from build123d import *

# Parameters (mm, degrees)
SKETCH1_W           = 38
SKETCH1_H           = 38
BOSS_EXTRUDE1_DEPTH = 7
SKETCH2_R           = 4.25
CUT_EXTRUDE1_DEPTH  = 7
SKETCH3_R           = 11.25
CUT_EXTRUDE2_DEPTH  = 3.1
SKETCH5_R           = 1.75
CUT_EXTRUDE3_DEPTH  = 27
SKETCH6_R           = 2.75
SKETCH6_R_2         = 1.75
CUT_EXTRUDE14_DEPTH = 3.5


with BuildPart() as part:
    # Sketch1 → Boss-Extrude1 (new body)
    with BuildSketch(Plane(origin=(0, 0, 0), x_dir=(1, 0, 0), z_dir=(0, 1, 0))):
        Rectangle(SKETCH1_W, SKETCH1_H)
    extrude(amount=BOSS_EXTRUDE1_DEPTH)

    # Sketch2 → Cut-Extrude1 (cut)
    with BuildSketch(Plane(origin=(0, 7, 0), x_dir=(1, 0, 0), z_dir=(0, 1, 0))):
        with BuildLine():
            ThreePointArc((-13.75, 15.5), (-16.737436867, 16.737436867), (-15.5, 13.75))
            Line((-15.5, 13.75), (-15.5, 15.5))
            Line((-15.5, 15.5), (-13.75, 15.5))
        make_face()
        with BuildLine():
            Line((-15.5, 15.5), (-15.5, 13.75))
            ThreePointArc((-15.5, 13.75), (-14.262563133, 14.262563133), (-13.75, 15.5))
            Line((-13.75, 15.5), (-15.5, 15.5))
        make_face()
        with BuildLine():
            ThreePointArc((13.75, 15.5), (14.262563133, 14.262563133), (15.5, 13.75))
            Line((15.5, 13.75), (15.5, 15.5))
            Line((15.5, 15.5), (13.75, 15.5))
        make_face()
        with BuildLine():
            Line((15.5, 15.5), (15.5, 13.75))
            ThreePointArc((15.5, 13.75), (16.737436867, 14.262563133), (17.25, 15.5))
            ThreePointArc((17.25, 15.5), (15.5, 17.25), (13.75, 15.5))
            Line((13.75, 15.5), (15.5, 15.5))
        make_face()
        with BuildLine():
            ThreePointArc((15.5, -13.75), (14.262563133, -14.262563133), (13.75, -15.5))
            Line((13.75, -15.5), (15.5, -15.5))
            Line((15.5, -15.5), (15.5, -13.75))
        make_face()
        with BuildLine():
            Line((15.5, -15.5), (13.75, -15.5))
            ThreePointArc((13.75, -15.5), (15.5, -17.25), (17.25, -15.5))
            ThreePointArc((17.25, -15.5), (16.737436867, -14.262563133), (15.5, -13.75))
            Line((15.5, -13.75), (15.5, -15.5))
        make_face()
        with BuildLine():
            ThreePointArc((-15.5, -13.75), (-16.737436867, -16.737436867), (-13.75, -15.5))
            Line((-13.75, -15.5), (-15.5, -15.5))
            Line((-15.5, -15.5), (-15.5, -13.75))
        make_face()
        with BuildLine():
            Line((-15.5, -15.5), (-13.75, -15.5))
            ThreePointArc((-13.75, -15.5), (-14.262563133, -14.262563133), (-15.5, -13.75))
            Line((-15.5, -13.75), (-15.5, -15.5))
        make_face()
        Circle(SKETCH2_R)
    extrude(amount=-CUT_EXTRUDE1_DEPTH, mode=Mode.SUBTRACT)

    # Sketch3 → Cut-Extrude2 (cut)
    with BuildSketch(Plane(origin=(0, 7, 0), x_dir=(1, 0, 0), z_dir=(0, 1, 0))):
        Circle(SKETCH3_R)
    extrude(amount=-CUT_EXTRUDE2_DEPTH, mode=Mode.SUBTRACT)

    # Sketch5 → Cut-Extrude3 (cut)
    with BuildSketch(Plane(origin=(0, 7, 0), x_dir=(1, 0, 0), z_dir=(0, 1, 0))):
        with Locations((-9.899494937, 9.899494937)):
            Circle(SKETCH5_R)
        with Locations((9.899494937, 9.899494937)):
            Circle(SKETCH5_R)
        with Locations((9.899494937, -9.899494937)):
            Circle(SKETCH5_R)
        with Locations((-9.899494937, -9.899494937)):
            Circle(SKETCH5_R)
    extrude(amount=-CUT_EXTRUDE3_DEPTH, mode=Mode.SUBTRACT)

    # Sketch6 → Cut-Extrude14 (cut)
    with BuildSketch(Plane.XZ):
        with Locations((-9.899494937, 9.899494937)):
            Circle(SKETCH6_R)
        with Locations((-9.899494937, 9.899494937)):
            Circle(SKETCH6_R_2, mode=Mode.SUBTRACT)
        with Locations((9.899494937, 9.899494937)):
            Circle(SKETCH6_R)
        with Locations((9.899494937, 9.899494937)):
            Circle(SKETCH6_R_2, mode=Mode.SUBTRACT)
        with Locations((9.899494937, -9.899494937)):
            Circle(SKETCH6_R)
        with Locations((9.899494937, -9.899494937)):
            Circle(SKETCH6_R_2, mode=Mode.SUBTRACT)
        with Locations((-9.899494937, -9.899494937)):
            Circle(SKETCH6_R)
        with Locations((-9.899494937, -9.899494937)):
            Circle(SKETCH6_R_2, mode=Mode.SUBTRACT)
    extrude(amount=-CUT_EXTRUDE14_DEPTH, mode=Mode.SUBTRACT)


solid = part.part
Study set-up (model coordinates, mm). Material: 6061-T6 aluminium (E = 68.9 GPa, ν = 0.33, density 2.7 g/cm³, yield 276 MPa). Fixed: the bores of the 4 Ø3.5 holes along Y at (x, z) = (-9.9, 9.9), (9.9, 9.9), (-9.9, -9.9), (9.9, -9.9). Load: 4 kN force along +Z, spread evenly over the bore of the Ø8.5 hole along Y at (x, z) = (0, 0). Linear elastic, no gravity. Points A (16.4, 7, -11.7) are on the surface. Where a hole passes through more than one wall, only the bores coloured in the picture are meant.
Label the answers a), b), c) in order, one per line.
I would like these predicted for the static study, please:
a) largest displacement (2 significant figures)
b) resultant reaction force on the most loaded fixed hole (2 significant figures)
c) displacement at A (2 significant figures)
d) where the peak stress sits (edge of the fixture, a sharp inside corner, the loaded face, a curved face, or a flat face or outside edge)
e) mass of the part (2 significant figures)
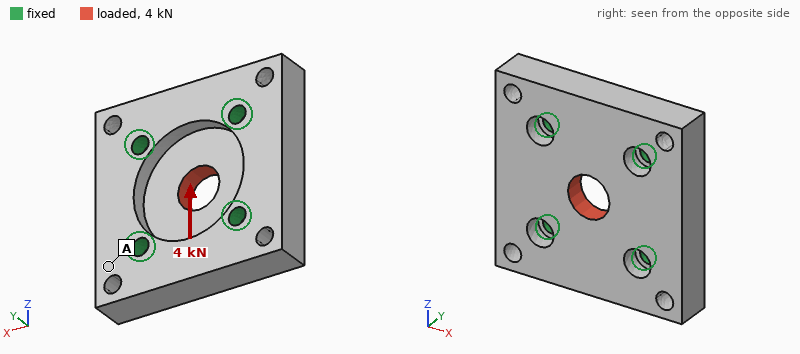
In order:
a) 9.7 µm
b) 1.0 kN
c) 1.6 µm
d) edge of the fixture
e) 21 g
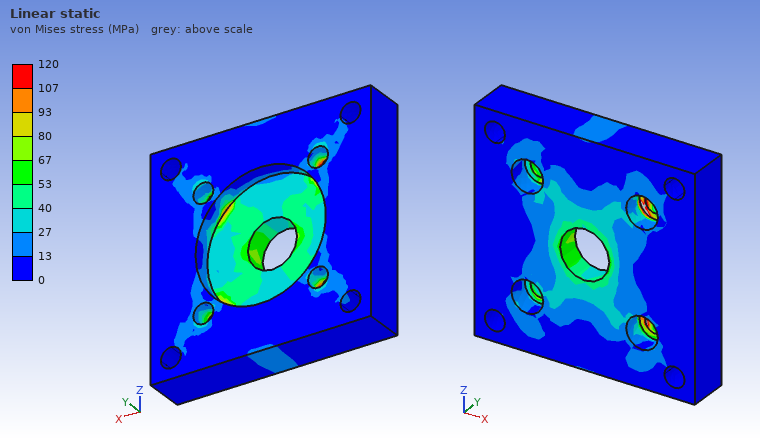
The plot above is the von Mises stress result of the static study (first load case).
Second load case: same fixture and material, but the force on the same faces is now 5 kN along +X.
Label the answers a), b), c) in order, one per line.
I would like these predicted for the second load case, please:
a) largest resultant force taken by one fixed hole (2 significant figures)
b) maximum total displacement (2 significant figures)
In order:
a) 1.3 kN
b) 12 µm
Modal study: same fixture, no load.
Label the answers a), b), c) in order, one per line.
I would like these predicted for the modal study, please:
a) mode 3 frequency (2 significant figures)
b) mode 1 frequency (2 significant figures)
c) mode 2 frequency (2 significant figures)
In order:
a) 28 kHz
b) 28 kHz
c) 28 kHz
